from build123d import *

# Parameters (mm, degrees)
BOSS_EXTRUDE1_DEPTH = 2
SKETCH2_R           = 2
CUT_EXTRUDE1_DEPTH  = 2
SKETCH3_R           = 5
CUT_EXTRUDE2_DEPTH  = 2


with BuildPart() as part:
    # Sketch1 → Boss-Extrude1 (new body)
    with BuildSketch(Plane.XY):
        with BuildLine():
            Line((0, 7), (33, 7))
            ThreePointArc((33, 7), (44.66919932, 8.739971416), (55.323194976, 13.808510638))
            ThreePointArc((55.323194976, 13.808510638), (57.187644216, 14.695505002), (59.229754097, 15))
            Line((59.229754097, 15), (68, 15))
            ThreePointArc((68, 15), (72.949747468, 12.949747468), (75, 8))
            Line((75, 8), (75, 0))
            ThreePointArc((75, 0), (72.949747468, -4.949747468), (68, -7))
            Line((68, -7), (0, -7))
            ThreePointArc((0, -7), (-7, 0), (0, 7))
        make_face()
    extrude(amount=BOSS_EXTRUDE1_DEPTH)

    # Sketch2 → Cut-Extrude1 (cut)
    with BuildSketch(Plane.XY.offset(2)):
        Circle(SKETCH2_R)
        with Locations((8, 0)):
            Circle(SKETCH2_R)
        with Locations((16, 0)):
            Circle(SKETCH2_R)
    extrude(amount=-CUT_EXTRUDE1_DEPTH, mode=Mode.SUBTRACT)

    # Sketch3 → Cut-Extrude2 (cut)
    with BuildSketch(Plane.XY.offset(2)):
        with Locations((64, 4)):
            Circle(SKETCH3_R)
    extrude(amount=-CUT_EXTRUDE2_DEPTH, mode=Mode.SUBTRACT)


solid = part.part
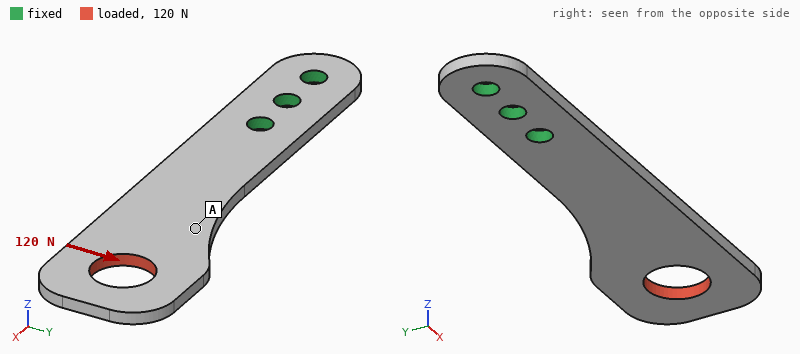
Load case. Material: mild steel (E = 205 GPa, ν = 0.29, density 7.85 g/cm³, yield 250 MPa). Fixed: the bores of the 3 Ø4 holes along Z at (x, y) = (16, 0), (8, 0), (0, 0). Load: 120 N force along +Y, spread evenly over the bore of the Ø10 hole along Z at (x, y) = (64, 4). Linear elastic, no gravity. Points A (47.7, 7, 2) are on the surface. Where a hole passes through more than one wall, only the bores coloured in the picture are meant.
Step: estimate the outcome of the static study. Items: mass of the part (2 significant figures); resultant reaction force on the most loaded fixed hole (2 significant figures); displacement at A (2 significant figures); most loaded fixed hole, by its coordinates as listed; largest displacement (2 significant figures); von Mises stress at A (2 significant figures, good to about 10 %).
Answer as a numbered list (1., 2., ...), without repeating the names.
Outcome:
1. 19 g
2. 410 N
3. 35 µm
4. (16, 0)
5. 80 µm
6. 14 MPa
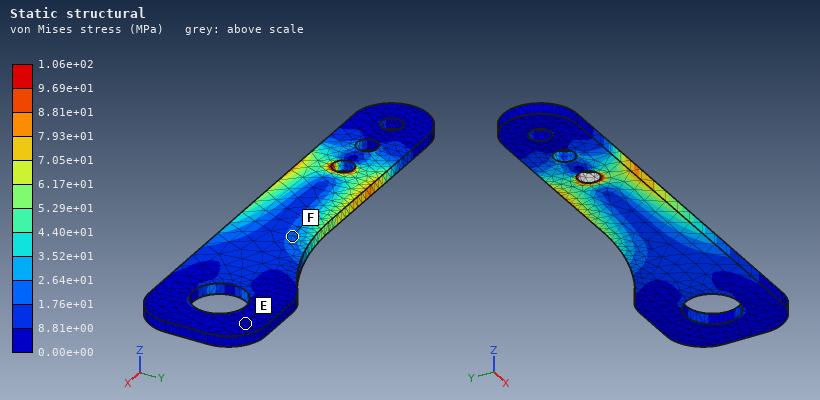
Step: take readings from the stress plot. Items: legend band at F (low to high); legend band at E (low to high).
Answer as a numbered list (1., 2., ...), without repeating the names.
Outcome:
1. 1.76e+01 to 2.64e+01 MPa
2. 0.00e+00 to 8.81e+00 MPa
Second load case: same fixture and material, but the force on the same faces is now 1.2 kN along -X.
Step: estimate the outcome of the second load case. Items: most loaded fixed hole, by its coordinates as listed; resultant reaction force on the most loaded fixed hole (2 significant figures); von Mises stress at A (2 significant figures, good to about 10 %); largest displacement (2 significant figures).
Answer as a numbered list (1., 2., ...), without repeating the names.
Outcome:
1. (16, 0)
2. 1.0 kN
3. 59 MPa
4. 86 µm
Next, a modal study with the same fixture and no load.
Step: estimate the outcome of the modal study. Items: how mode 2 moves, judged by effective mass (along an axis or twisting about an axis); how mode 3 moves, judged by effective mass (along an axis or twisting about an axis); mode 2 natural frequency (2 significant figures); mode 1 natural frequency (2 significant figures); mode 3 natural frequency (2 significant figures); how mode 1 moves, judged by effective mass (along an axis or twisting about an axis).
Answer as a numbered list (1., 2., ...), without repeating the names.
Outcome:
1. twisting about X
2. along Y
3. 2400 Hz
4. 450 Hz
5. 2600 Hz
6. along Z
